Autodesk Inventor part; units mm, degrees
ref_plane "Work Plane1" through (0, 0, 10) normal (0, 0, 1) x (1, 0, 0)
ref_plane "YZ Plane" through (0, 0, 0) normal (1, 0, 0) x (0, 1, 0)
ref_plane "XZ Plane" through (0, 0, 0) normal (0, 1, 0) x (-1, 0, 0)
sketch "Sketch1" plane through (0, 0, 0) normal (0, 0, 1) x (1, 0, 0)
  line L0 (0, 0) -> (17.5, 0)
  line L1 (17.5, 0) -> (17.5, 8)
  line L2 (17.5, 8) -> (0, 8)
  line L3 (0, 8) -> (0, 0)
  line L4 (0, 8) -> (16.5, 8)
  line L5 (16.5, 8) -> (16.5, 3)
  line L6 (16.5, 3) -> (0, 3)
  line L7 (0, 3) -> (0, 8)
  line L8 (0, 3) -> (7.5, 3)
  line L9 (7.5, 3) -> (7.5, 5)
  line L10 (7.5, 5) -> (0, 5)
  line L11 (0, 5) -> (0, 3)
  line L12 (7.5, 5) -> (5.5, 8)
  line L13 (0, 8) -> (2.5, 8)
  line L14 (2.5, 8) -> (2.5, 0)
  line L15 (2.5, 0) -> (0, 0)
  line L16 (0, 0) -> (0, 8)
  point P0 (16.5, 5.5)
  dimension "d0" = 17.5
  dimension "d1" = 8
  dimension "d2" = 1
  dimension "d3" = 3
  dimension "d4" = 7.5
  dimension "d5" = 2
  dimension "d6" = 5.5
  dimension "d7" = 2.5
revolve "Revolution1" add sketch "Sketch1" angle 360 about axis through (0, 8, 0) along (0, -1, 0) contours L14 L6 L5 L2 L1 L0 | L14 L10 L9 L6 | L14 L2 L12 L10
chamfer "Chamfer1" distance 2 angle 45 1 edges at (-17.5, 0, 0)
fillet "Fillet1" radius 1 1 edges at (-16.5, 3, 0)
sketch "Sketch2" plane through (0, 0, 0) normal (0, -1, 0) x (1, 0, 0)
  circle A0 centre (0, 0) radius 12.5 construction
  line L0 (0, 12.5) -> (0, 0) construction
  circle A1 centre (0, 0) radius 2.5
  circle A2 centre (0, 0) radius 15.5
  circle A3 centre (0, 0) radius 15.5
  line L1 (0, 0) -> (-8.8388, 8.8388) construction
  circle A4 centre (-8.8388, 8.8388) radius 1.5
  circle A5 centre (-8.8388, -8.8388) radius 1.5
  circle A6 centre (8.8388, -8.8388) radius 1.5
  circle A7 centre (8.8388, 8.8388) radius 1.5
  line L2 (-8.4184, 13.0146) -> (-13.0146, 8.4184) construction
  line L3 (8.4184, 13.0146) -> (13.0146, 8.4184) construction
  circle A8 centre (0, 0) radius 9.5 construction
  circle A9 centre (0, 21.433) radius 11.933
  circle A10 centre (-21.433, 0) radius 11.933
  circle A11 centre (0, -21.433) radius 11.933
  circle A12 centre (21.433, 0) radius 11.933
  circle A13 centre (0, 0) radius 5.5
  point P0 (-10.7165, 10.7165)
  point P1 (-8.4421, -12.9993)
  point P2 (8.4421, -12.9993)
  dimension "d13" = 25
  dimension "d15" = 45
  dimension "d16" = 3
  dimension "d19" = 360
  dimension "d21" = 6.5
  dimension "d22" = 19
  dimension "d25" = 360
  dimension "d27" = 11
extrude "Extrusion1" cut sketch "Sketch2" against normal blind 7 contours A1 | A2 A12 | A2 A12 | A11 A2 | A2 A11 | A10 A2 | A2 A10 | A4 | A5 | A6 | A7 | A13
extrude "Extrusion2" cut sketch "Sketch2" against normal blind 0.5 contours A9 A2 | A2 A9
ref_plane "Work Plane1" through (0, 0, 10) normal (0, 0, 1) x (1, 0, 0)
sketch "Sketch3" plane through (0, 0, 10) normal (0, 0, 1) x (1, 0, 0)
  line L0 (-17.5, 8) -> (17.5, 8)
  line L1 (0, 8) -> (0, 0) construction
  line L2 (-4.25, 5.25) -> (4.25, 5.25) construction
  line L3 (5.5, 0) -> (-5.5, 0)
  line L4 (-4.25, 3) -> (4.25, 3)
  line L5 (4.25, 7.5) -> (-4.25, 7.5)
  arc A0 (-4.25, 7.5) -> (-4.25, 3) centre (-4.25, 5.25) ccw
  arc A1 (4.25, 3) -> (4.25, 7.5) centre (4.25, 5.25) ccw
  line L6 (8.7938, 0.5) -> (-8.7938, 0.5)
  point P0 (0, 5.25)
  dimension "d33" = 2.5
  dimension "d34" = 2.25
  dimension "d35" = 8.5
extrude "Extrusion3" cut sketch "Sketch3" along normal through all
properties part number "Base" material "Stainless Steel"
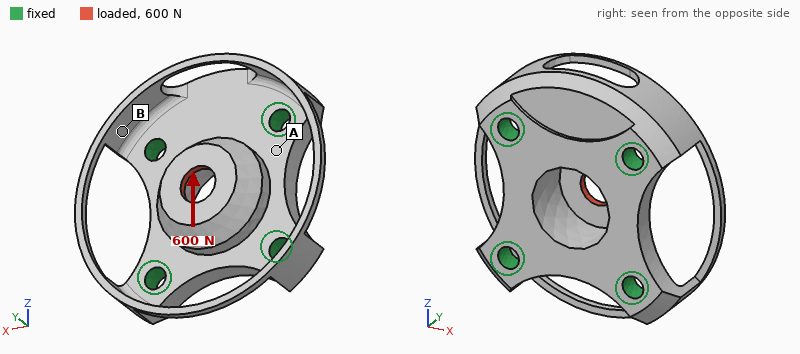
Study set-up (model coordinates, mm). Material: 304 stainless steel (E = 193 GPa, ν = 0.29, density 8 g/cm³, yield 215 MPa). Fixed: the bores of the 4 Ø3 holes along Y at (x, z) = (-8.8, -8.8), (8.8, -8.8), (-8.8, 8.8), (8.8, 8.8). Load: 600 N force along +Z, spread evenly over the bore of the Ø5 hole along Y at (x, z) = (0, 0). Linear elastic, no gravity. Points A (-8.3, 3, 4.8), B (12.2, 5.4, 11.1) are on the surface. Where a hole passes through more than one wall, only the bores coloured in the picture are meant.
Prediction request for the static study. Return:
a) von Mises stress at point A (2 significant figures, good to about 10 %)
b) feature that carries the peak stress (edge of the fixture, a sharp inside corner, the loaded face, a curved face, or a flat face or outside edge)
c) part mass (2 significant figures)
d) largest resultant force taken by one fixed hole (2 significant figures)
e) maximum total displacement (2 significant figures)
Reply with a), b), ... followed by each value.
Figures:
a) 14 MPa
b) the loaded face
c) 16 g
d) 200 N
e) 4.3 µm
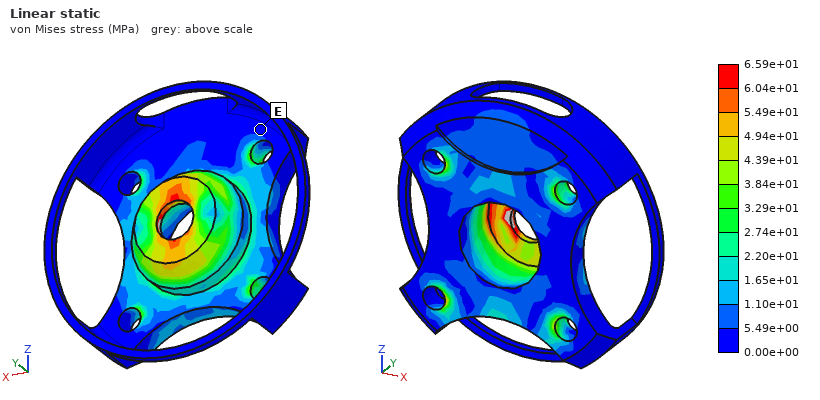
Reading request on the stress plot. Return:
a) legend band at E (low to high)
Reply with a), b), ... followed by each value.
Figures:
a) 0.00e+00 to 5.49e+00 MPa
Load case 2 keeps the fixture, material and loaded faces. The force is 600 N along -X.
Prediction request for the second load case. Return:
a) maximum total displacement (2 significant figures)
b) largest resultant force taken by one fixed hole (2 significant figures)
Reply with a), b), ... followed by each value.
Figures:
a) 4.4 µm
b) 210 N
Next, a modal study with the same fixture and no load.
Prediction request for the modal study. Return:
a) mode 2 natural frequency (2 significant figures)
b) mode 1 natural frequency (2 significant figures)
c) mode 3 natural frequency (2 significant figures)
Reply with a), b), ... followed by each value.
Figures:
a) 10 kHz
b) 10 kHz
c) 10 kHz
